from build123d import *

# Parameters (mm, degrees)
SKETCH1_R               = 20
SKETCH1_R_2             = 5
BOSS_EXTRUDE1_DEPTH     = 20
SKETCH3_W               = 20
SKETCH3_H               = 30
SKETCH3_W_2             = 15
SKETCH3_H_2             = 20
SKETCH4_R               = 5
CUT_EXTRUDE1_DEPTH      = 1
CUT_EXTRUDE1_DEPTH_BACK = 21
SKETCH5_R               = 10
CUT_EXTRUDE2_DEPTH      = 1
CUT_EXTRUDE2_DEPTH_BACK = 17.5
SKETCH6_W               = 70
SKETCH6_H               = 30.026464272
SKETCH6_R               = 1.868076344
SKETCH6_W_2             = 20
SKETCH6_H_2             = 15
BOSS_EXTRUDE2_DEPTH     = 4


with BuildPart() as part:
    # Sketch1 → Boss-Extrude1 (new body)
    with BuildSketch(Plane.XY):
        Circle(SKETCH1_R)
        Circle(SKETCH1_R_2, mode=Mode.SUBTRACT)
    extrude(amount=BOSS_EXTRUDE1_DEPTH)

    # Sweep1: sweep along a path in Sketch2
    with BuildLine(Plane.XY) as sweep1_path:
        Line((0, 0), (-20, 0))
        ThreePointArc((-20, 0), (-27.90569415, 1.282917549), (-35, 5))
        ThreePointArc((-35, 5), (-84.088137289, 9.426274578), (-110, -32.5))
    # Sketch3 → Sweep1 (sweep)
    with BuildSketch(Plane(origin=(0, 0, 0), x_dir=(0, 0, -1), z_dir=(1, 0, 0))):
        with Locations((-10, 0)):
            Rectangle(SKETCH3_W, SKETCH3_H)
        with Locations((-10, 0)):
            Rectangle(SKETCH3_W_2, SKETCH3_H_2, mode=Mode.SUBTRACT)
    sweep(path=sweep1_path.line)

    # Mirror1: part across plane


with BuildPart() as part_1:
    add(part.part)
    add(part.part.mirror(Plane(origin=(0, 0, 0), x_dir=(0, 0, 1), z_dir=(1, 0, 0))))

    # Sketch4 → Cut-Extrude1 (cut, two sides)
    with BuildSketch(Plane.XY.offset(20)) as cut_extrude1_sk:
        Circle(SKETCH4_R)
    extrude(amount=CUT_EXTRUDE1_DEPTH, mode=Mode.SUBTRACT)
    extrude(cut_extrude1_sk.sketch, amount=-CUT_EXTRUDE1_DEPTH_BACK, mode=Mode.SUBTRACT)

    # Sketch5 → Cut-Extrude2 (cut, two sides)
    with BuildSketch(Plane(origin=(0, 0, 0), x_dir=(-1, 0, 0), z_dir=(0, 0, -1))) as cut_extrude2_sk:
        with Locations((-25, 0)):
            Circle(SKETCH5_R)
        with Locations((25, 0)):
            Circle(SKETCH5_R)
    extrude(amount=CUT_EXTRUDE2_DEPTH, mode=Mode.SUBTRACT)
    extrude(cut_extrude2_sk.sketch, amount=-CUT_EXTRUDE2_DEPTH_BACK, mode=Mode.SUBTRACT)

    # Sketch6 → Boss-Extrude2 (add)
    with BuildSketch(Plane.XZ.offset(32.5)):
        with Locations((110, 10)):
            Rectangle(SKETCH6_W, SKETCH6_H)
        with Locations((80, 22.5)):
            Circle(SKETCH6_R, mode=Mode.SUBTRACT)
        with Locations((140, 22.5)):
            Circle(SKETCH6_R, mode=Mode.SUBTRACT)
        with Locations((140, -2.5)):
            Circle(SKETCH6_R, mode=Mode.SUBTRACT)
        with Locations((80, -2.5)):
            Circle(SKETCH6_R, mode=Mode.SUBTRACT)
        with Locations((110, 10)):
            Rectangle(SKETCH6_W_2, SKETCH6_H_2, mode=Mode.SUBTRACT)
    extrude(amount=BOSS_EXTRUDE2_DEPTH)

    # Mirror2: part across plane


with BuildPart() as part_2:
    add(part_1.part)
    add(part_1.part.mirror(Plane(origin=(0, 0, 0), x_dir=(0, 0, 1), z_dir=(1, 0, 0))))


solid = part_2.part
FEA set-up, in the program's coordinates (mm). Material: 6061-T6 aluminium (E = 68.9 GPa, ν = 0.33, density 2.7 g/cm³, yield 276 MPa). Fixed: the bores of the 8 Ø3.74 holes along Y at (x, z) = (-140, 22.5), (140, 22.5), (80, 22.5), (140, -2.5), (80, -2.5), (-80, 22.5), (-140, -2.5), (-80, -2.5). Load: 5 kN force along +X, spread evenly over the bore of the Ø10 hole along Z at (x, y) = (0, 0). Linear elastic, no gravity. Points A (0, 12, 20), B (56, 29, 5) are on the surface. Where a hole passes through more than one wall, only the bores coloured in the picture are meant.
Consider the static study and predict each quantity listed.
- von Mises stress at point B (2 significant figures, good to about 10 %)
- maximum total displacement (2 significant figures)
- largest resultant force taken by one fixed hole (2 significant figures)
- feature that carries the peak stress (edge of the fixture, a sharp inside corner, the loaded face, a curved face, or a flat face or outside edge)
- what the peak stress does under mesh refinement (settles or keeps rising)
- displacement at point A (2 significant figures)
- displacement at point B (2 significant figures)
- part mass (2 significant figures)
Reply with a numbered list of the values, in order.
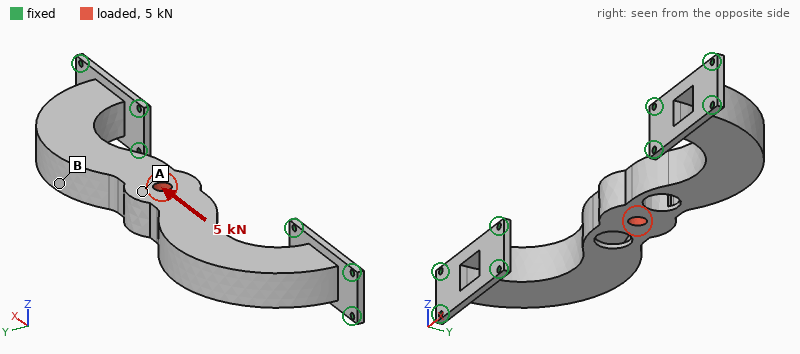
1. 18 MPa
2. 0.13 mm
3. 860 N
4. edge of the fixture
5. keeps rising
6. 0.10 mm
7. 0.11 mm
8. 290 g
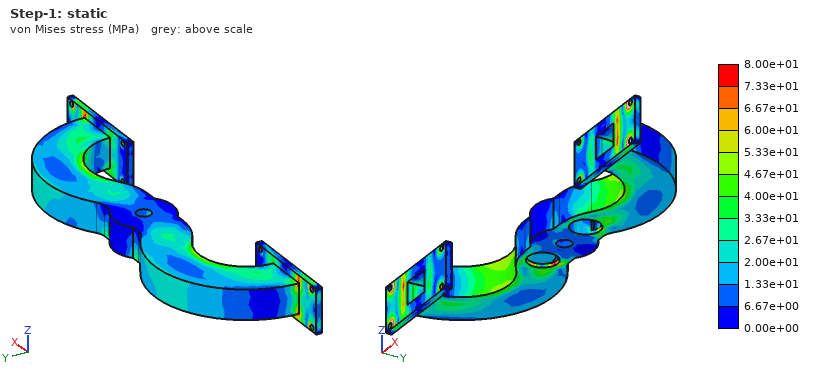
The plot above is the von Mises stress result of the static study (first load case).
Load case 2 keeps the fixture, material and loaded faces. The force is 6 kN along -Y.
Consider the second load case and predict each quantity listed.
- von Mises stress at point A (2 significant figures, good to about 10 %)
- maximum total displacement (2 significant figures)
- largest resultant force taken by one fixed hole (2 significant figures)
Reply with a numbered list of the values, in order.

1. 52 MPa
2. 0.40 mm
3. 1.3 kN
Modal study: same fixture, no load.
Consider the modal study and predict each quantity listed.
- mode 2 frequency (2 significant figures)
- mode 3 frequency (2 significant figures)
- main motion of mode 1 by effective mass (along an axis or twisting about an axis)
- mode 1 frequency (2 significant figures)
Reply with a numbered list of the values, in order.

1. 1800 Hz
2. 1800 Hz
3. along Z
4. 680 Hz
